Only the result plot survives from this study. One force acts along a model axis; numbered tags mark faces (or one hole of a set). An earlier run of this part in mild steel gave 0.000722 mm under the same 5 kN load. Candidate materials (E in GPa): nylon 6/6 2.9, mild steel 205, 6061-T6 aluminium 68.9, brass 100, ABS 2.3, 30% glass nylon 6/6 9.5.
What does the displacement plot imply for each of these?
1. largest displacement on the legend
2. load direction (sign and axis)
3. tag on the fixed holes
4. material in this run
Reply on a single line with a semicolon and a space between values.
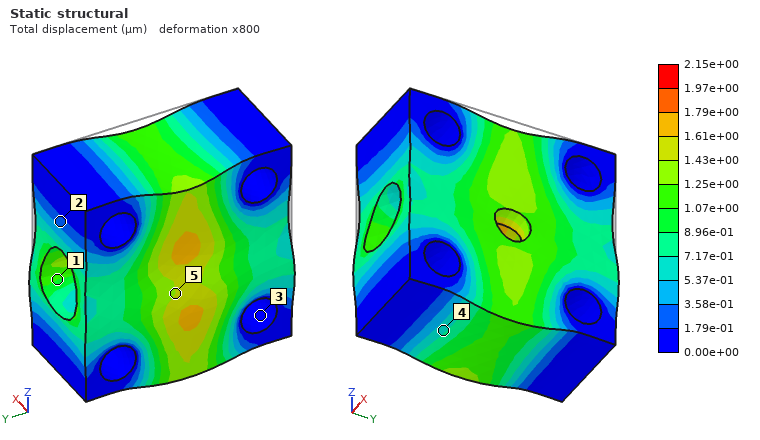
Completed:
2.15e+00 µm; -Z; 3; 6061-T6 aluminium
